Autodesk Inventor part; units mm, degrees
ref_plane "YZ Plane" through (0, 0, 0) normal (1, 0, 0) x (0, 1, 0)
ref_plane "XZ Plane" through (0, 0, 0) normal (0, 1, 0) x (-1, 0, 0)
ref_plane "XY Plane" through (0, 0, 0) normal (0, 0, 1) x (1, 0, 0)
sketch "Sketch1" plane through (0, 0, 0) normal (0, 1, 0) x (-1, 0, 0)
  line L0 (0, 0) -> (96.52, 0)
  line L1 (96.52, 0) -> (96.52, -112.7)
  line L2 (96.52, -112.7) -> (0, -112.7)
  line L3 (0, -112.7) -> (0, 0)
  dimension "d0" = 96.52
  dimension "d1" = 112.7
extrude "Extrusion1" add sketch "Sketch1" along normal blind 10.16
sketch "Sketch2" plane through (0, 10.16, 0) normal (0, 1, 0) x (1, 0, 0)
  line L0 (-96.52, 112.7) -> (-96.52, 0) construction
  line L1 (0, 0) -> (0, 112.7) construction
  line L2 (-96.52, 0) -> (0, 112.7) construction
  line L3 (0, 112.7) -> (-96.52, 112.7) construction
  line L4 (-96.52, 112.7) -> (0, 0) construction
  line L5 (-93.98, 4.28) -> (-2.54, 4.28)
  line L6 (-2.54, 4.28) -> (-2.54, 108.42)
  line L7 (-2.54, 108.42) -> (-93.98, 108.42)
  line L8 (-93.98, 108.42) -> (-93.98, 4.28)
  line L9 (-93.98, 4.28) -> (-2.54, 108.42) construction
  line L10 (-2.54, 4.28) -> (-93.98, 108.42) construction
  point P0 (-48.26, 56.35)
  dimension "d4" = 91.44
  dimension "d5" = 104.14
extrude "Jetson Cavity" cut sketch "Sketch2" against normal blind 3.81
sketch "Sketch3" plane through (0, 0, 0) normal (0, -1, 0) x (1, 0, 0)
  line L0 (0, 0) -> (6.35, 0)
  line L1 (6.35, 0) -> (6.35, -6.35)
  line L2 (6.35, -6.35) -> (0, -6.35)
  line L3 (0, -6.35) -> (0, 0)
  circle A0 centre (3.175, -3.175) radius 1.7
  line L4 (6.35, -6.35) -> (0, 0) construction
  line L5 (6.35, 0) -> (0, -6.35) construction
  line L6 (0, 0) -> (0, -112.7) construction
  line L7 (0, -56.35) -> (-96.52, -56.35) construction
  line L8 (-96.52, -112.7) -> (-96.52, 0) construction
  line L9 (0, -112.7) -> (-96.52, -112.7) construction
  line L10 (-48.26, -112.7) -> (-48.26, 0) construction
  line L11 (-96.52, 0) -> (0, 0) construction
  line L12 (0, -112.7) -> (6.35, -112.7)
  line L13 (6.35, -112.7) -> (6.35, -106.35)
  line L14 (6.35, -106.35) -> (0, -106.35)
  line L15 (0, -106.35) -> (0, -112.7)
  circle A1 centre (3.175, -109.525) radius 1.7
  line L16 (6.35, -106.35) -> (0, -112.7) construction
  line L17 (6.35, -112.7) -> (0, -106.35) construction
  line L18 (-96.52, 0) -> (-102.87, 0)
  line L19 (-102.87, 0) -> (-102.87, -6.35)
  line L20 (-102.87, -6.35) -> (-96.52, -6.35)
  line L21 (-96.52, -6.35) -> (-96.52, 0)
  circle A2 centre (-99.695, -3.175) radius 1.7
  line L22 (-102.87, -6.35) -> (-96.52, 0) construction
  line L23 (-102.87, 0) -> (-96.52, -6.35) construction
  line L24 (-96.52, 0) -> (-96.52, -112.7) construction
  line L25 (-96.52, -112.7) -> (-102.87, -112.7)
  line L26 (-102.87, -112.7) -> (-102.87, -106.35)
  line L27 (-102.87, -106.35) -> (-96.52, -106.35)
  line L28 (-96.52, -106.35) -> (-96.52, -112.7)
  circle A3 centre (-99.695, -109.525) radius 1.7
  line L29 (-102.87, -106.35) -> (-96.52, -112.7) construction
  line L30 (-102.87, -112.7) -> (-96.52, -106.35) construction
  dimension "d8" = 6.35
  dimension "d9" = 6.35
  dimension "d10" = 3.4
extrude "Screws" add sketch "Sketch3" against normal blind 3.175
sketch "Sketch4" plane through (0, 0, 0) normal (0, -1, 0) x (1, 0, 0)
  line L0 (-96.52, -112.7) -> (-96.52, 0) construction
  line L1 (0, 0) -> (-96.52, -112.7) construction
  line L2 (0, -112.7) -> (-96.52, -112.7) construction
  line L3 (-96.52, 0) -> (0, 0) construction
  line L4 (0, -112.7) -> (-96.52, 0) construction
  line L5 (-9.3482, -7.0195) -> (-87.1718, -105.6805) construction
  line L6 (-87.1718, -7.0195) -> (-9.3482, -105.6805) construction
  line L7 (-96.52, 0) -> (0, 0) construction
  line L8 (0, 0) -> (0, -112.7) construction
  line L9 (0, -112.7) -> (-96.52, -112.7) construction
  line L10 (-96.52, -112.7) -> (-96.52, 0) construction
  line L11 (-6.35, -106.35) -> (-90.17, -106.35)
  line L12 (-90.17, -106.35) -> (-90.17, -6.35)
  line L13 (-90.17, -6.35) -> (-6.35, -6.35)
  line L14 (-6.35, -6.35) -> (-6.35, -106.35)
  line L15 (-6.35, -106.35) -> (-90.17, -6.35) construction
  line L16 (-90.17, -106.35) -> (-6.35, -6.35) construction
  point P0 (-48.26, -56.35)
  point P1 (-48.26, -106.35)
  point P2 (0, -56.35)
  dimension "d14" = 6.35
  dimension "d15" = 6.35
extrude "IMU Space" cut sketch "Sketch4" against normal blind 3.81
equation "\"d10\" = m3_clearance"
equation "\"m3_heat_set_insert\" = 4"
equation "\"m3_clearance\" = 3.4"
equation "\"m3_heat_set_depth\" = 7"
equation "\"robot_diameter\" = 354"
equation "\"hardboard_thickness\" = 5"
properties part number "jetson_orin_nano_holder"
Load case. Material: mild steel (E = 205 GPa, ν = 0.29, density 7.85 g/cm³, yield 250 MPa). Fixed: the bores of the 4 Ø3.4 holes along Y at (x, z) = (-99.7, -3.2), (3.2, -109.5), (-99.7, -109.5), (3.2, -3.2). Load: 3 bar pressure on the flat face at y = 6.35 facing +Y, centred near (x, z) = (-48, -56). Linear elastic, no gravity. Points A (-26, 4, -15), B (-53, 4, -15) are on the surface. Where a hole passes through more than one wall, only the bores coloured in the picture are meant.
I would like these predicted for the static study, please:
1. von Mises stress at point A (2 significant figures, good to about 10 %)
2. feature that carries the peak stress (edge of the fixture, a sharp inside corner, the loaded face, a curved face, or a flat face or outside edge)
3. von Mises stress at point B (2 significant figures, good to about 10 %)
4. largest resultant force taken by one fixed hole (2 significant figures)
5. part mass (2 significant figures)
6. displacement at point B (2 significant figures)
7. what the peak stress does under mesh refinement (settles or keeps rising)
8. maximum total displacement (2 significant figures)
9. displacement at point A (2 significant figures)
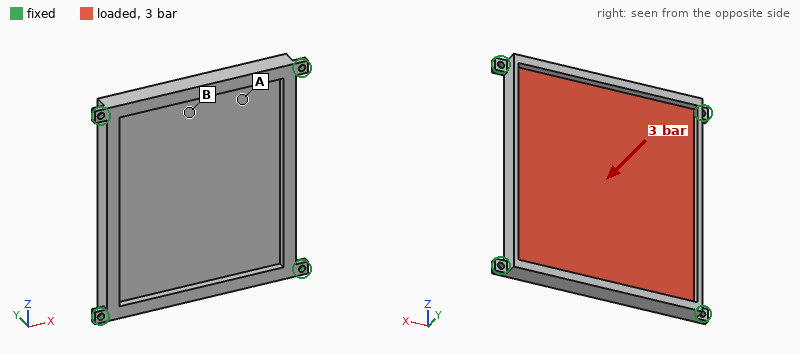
49 MPa
edge of the fixture
21 MPa
2.7 kN
340 g
0.13 mm
keeps rising
0.31 mm
0.10 mm
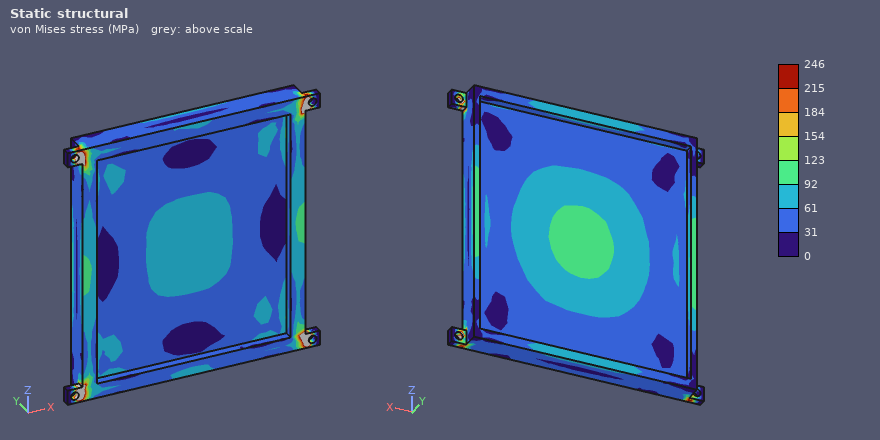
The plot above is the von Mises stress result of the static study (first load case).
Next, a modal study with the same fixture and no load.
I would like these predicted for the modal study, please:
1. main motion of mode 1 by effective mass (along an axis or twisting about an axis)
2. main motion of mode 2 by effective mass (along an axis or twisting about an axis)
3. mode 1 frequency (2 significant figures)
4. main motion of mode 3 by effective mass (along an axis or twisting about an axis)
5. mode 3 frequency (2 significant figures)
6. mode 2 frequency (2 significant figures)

along Y
twisting about Z
1300 Hz
twisting about X
2500 Hz
2200 Hz
